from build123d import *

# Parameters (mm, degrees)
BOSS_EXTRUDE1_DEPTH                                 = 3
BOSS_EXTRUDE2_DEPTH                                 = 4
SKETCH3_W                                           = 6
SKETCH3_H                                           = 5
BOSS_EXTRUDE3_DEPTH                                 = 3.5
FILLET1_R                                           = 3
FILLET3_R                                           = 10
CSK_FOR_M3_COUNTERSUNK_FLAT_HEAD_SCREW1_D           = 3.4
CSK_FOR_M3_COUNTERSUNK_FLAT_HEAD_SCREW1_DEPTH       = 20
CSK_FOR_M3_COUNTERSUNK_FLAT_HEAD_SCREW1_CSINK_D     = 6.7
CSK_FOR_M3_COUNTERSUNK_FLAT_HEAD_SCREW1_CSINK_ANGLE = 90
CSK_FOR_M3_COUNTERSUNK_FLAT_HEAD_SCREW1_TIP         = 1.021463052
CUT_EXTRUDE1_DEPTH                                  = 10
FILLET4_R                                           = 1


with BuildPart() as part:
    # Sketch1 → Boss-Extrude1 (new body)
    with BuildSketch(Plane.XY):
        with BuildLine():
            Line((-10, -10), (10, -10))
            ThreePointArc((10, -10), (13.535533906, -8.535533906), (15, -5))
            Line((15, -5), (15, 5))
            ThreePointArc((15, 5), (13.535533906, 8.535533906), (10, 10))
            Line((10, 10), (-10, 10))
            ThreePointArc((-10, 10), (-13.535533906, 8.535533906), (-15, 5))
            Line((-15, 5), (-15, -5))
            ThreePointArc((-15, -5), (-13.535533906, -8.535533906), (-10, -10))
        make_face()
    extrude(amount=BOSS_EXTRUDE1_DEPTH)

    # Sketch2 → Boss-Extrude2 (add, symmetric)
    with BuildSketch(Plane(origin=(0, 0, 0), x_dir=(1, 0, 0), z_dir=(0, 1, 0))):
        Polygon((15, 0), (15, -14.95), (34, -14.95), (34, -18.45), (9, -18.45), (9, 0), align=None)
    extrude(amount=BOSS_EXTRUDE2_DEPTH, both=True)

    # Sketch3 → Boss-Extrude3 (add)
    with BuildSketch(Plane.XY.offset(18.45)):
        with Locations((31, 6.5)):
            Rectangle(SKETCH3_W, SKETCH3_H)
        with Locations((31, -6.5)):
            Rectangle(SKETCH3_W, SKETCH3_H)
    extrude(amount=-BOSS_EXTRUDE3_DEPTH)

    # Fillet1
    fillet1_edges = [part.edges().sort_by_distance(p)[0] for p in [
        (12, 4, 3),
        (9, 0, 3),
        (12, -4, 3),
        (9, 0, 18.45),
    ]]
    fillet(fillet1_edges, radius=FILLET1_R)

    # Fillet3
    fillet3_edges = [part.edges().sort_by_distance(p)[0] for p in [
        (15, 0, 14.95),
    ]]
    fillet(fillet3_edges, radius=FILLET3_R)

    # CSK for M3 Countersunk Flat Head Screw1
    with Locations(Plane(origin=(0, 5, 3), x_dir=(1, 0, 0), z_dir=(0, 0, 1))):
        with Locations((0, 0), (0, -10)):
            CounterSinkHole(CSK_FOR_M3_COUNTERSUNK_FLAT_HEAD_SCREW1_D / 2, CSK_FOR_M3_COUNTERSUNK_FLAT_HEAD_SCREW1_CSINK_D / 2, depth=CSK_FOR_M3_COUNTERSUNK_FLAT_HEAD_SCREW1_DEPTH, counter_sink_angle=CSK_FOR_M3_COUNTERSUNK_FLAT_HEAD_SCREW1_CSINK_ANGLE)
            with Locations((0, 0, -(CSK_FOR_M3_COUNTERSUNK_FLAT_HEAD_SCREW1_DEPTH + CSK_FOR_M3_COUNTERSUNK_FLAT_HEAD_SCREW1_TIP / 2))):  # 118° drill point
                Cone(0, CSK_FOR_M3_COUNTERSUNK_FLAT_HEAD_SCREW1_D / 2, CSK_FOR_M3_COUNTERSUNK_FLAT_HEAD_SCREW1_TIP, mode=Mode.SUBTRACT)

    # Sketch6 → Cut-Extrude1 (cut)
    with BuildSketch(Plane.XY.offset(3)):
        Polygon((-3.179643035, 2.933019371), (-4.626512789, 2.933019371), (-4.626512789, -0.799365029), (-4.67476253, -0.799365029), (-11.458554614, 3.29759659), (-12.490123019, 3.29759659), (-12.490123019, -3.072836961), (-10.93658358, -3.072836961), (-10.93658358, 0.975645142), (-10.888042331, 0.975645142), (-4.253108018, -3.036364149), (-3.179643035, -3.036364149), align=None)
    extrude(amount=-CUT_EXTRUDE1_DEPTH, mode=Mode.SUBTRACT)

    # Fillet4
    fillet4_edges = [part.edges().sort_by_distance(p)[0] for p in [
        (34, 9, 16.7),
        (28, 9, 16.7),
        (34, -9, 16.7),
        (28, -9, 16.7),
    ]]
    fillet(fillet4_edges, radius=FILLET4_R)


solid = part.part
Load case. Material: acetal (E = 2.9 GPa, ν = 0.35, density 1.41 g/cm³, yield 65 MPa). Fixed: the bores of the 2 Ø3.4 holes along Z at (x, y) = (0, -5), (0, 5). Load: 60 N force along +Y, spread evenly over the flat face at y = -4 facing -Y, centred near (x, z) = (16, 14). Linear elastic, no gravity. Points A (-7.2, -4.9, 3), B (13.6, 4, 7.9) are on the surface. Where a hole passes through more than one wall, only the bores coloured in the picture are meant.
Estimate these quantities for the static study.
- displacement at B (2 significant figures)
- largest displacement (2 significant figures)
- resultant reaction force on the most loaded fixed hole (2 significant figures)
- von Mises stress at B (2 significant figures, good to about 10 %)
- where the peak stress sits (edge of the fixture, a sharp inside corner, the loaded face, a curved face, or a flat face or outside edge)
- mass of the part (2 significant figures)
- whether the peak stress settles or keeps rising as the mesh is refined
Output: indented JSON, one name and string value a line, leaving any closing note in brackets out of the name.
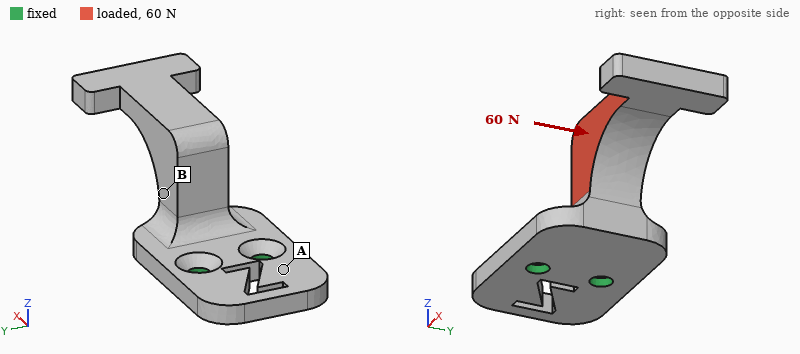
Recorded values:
{
  "displacement at B": "0.18 mm",
  "largest displacement": "0.55 mm",
  "resultant reaction force on the most loaded fixed hole": "110 N",
  "von Mises stress at B": "6.8 MPa",
  "where the peak stress sits": "edge of the fixture",
  "mass of the part": "4.6 g",
  "whether the peak stress settles or keeps rising as the mesh is refined": "keeps rising"
}
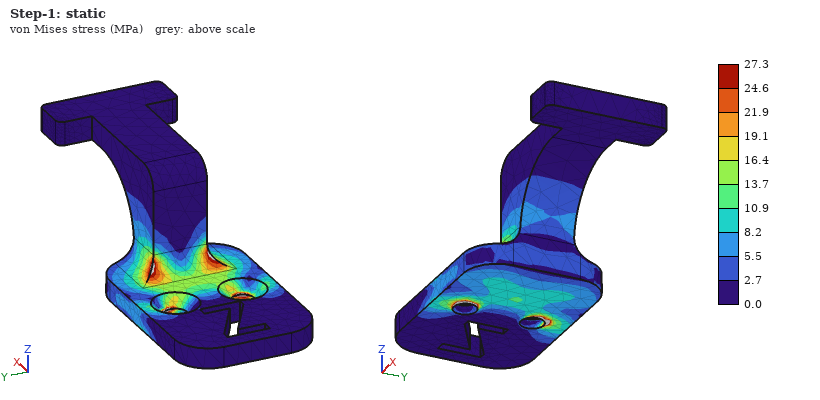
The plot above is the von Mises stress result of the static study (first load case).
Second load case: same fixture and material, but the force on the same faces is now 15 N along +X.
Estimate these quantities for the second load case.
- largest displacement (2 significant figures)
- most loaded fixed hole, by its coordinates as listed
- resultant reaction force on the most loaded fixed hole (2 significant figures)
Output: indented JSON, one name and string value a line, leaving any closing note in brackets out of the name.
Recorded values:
{
  "largest displacement": "0.64 mm",
  "most loaded fixed hole, by its coordinates as listed": "(0, -5)",
  "resultant reaction force on the most loaded fixed hole": "13 N"
}
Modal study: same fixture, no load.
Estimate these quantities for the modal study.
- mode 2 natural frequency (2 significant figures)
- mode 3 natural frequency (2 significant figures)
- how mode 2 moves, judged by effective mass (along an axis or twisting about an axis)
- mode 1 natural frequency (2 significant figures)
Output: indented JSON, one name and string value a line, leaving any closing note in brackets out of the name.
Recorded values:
{
  "mode 2 natural frequency": "1200 Hz",
  "mode 3 natural frequency": "2400 Hz",
  "how mode 2 moves, judged by effective mass": "along Y",
  "mode 1 natural frequency": "480 Hz"
}
